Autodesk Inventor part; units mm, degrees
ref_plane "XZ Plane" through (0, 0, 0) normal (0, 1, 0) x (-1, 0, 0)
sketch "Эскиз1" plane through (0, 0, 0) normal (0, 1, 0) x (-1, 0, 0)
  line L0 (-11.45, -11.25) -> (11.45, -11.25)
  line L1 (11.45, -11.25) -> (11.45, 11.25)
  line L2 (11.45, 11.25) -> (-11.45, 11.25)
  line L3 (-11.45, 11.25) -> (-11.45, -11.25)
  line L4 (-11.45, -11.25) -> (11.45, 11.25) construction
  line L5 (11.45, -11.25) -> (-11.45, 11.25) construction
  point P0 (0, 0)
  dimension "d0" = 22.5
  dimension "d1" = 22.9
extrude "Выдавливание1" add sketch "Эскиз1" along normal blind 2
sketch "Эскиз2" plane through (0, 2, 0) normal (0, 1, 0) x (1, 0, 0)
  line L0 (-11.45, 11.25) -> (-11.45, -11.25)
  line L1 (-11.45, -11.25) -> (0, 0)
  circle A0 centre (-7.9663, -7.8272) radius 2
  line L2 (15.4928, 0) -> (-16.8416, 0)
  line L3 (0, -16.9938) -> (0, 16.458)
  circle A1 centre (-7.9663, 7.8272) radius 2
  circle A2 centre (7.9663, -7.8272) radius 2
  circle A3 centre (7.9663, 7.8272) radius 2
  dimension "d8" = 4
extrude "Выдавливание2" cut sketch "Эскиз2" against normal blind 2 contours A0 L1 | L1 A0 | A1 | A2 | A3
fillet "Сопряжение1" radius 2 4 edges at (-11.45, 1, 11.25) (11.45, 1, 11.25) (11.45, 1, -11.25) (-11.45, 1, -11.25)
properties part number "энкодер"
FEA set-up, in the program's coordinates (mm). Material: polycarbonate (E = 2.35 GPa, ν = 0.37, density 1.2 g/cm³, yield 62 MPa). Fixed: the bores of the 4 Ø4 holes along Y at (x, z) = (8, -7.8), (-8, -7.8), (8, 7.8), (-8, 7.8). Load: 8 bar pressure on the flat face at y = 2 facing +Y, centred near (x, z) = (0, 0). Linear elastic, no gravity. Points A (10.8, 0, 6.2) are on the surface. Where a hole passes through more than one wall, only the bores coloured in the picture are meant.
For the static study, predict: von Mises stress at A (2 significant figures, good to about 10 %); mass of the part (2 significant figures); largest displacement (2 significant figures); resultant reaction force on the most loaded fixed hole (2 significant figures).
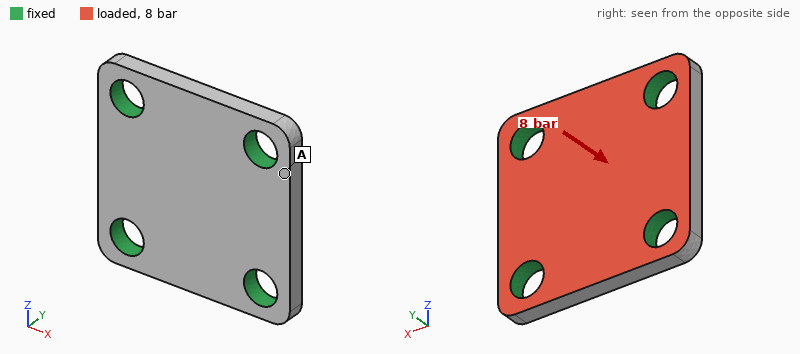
5.8 MPa
1.1 g
0.11 mm
92 N
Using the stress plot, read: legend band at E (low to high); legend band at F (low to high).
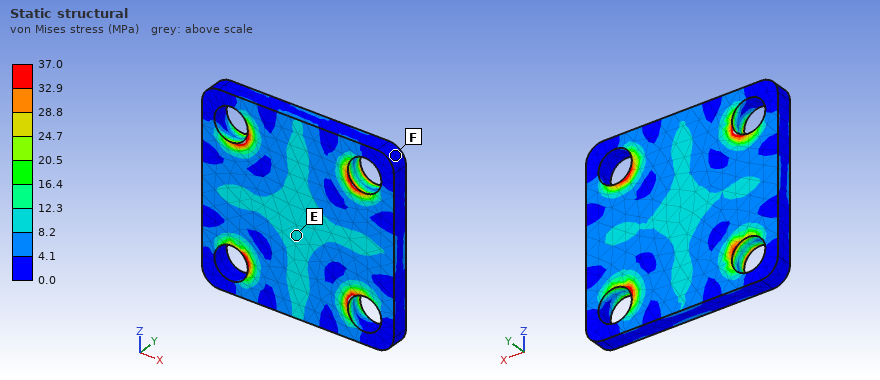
8.2 to 12.3 MPa
0.0 to 4.1 MPa
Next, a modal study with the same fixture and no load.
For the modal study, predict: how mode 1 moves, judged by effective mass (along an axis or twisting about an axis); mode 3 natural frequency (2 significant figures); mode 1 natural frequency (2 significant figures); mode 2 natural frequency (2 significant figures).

along Y
16 kHz
11 kHz
16 kHz
